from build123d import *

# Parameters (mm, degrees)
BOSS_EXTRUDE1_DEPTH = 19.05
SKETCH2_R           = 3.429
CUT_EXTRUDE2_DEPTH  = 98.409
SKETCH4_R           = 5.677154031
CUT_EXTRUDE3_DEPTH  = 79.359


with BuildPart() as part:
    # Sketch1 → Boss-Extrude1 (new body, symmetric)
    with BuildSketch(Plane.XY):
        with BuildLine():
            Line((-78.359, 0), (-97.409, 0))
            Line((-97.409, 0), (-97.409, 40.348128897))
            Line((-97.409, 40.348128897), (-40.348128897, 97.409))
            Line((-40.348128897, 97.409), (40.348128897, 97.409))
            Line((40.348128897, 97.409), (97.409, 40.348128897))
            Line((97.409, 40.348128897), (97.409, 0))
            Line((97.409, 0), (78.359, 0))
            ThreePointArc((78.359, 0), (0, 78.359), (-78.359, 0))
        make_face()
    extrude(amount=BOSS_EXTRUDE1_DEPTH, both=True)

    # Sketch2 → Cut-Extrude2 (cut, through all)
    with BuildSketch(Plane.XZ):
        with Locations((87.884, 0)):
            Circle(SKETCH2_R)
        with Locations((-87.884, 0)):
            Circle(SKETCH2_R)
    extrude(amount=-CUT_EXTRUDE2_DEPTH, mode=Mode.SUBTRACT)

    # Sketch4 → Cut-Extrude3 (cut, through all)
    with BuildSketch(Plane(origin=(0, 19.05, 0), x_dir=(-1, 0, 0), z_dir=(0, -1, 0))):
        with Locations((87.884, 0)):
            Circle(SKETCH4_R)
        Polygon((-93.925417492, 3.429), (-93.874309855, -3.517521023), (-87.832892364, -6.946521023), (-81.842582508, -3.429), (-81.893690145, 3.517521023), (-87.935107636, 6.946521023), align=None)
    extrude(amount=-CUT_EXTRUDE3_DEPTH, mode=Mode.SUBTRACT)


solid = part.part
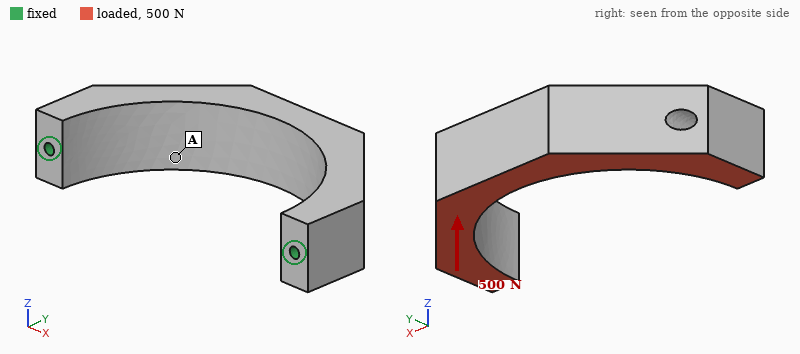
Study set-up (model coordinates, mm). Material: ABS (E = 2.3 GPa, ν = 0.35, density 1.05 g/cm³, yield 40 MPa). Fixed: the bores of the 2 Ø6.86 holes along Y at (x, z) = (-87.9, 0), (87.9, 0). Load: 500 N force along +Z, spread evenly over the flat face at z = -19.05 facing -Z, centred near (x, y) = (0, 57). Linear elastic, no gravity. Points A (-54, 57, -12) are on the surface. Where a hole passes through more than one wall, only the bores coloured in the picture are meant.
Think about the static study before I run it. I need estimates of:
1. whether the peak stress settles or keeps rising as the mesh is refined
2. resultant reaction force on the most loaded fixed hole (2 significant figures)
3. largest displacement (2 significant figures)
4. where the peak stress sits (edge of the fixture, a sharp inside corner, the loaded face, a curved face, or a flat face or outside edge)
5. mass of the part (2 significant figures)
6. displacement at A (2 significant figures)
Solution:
keeps rising
250 N
0.45 mm
edge of the fixture
230 g
0.22 mm
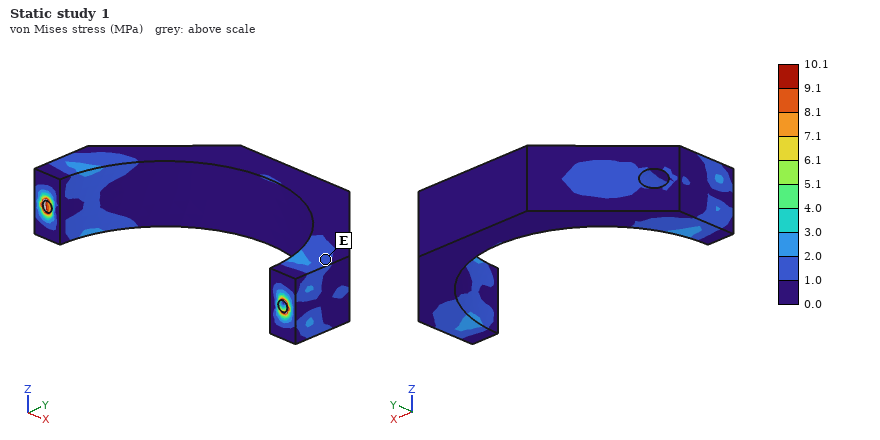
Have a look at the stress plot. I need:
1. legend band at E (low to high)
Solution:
1.0 to 2.0 MPa
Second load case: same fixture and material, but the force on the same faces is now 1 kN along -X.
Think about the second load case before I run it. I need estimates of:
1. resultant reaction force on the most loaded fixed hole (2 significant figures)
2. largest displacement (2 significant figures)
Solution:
530 N
0.26 mm
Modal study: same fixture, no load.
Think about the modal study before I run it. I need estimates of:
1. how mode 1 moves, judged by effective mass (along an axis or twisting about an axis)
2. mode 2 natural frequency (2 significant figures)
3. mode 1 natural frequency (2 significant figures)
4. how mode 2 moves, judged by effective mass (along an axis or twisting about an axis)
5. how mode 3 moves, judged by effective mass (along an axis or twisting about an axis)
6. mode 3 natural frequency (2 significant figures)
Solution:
along Z
740 Hz
400 Hz
along X
twisting about Y
1100 Hz
